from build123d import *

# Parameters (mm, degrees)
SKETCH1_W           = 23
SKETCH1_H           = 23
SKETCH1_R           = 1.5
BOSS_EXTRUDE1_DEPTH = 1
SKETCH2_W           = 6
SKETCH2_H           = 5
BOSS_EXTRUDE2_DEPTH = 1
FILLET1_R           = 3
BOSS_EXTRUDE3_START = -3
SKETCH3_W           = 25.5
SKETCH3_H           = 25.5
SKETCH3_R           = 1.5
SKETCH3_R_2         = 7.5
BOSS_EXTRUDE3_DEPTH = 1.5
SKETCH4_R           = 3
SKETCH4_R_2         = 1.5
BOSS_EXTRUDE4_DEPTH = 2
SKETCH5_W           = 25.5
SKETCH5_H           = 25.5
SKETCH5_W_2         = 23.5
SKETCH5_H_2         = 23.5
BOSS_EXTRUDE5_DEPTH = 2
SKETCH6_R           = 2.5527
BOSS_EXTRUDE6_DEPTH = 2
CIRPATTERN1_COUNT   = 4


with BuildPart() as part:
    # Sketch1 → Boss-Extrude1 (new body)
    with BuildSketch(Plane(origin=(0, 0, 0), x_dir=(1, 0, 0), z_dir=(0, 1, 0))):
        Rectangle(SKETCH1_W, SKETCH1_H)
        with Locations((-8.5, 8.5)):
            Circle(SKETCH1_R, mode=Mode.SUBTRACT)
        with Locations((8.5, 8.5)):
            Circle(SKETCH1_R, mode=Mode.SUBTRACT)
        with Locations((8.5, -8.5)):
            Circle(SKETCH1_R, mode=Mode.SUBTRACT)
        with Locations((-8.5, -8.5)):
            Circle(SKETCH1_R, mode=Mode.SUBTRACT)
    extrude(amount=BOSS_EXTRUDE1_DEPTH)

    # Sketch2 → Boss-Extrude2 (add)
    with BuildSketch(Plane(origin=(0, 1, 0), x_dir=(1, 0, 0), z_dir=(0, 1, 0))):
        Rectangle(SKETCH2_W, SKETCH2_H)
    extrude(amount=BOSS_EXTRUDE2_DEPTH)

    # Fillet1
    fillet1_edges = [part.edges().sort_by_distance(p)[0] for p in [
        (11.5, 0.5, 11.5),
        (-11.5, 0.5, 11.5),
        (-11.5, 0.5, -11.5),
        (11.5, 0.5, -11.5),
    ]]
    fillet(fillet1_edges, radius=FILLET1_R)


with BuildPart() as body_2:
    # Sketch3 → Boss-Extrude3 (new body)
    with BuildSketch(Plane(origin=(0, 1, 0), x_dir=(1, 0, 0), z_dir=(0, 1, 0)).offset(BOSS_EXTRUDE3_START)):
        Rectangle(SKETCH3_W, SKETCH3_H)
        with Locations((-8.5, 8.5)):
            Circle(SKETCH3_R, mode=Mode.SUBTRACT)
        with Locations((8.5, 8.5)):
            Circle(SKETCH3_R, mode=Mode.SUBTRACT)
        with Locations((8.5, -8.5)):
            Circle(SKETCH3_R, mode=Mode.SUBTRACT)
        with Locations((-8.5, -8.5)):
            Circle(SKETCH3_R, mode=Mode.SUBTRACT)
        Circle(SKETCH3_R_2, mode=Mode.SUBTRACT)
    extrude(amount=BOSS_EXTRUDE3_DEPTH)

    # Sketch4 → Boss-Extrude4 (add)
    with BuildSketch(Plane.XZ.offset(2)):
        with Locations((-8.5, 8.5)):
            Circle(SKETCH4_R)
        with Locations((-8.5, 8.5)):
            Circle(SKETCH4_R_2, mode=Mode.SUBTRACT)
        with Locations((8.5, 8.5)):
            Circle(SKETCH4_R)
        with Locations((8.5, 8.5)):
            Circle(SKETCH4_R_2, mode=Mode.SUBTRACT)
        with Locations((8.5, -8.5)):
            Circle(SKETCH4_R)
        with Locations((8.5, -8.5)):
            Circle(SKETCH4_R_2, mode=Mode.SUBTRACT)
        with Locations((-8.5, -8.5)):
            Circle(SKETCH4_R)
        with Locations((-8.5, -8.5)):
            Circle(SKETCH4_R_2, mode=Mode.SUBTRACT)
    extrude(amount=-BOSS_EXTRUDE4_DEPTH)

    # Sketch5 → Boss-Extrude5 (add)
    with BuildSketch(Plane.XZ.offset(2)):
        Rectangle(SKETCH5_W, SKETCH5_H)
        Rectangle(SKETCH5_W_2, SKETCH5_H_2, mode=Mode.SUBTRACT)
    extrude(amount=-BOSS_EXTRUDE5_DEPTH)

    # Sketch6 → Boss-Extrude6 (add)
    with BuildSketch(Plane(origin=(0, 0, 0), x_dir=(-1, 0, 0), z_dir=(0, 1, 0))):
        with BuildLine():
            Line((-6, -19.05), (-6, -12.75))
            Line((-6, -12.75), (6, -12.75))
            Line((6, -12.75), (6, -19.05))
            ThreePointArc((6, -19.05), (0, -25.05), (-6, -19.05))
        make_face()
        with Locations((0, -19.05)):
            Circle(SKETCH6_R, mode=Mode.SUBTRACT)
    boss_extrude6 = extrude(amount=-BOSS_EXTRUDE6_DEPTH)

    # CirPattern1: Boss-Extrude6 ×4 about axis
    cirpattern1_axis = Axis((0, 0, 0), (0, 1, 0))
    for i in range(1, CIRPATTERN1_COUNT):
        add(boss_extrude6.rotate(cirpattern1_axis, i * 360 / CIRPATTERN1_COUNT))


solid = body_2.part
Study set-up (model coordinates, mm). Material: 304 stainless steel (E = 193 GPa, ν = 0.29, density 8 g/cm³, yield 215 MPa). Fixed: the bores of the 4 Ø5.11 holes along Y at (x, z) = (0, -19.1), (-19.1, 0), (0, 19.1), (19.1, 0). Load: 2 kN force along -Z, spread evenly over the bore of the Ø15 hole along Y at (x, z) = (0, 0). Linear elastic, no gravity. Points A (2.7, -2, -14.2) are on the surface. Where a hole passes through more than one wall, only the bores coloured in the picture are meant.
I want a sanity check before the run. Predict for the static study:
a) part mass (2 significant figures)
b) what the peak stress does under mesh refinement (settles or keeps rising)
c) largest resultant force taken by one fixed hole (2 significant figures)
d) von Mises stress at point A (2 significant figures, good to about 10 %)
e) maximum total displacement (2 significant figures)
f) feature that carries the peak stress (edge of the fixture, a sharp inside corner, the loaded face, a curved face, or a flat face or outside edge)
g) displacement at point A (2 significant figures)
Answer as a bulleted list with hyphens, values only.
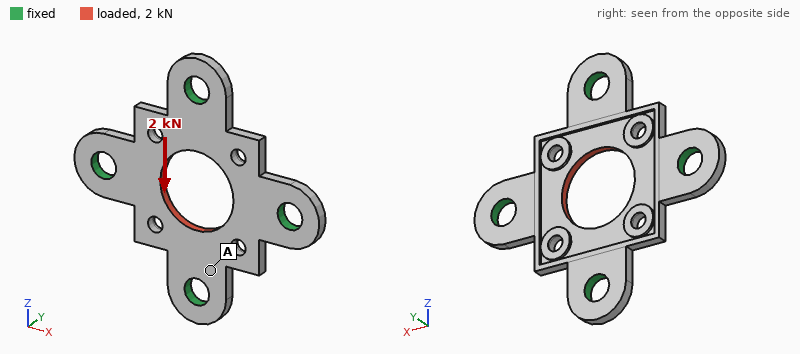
- 13 g
- keeps rising
- 740 N
- 39 MPa
- 3.7 µm
- edge of the fixture
- 0.84 µm
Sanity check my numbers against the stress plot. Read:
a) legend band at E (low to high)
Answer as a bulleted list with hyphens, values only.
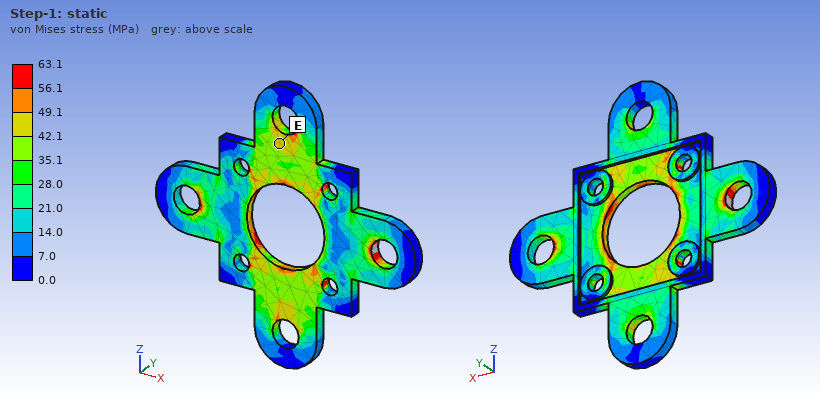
- 42.1 to 49.1 MPa
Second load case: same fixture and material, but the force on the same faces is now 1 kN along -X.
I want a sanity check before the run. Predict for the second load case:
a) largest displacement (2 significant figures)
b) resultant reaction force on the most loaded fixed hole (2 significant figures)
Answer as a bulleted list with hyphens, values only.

- 1.9 µm
- 370 N
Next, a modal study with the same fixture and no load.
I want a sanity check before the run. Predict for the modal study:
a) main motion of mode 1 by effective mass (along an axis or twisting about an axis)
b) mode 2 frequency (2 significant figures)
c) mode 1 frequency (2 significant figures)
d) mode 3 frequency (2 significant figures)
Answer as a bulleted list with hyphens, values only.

- along Y
- 18 kHz
- 16 kHz
- 18 kHz
